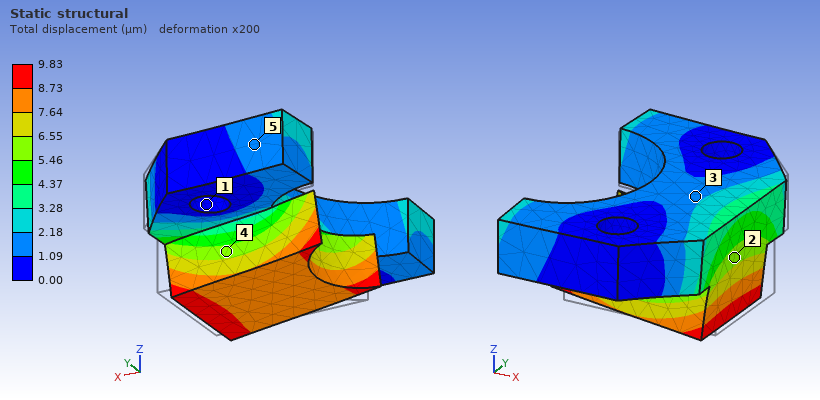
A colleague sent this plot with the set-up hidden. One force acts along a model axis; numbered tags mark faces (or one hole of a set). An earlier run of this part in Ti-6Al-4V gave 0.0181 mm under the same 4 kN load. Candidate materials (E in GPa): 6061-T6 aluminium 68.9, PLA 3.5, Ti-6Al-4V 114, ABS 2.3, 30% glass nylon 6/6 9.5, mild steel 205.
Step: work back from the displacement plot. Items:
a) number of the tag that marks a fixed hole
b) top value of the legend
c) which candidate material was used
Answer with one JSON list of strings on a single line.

["1", "9.83 µm", "mild steel"]
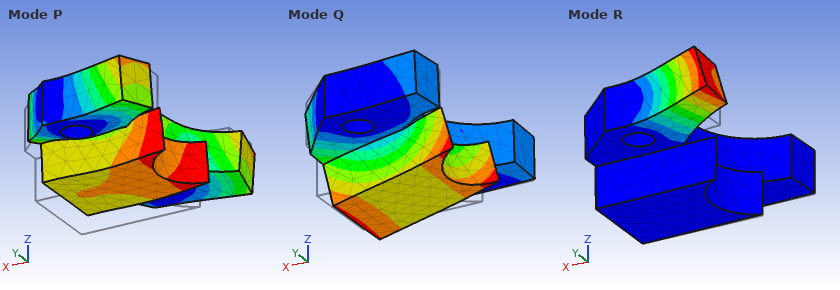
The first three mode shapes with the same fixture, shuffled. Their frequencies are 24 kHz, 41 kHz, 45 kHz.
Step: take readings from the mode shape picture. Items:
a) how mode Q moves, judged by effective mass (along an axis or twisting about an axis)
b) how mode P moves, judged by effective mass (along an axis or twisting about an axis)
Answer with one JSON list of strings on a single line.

["along X", "along Z"]
